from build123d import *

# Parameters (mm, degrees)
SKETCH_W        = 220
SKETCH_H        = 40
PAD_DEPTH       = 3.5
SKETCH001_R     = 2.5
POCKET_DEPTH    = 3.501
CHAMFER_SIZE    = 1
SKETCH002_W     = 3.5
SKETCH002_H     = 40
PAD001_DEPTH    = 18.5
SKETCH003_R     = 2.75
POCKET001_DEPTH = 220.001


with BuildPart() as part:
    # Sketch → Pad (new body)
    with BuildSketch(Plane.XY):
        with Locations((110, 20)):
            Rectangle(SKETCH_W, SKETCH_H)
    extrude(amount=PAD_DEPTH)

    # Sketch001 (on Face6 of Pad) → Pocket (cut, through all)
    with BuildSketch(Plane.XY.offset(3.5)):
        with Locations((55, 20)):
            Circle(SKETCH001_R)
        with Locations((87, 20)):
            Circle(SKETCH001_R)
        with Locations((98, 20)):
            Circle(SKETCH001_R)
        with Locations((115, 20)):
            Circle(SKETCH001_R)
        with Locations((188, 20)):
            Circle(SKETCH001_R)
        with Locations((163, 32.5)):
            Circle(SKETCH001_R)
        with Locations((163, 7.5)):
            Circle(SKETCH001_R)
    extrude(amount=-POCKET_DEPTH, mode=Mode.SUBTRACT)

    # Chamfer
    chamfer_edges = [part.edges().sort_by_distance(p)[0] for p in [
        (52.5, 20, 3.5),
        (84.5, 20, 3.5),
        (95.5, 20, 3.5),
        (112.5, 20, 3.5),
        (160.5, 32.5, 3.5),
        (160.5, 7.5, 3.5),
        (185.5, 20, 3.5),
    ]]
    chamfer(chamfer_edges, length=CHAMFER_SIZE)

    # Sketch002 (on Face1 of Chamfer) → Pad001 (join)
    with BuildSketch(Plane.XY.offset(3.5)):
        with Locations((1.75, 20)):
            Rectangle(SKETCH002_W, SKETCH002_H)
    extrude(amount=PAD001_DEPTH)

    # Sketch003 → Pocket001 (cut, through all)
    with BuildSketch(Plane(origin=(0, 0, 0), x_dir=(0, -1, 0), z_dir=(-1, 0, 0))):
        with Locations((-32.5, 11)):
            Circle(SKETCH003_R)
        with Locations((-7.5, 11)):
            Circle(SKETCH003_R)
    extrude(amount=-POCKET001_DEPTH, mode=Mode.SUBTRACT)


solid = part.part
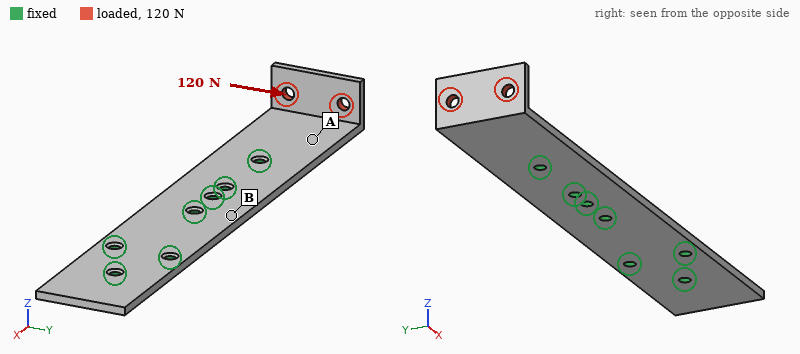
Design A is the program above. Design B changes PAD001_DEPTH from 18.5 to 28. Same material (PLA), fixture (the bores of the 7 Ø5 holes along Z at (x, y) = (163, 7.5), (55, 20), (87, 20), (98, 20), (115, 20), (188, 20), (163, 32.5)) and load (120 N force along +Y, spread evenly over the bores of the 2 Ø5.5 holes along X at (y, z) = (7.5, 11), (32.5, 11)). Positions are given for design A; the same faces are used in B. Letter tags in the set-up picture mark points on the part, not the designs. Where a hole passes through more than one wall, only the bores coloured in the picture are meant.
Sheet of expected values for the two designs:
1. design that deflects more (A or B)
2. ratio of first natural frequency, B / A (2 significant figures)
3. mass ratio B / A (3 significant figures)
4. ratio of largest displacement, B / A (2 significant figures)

B
0.84
1.04
1.2
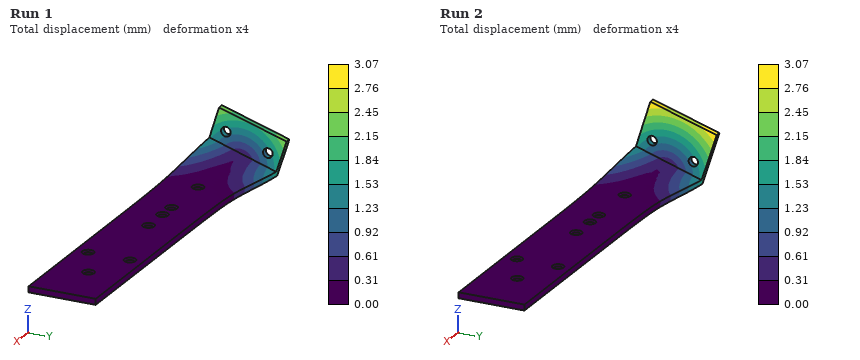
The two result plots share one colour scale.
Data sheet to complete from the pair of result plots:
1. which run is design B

Run 2
